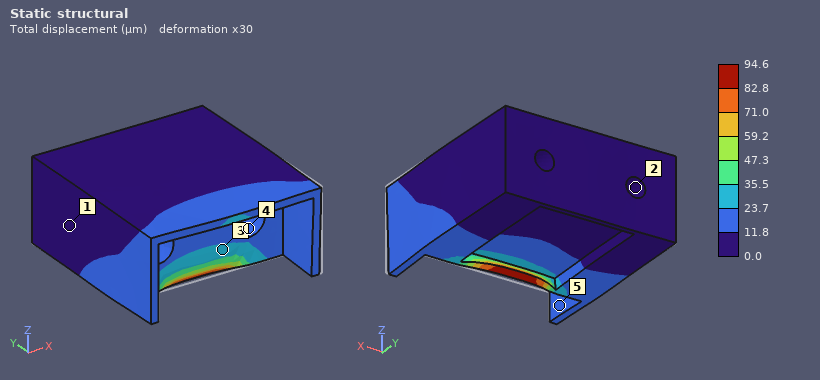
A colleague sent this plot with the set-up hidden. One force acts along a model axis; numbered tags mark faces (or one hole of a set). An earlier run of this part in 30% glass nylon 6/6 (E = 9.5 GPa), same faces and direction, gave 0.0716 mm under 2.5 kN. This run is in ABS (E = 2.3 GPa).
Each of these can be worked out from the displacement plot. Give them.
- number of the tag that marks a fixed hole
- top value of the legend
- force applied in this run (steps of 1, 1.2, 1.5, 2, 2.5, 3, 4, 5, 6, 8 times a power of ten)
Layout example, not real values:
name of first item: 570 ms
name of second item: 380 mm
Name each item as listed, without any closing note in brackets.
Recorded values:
number of the tag that marks a fixed hole: 2
top value of the legend: 94.6 µm
force applied in this run: 800 N
